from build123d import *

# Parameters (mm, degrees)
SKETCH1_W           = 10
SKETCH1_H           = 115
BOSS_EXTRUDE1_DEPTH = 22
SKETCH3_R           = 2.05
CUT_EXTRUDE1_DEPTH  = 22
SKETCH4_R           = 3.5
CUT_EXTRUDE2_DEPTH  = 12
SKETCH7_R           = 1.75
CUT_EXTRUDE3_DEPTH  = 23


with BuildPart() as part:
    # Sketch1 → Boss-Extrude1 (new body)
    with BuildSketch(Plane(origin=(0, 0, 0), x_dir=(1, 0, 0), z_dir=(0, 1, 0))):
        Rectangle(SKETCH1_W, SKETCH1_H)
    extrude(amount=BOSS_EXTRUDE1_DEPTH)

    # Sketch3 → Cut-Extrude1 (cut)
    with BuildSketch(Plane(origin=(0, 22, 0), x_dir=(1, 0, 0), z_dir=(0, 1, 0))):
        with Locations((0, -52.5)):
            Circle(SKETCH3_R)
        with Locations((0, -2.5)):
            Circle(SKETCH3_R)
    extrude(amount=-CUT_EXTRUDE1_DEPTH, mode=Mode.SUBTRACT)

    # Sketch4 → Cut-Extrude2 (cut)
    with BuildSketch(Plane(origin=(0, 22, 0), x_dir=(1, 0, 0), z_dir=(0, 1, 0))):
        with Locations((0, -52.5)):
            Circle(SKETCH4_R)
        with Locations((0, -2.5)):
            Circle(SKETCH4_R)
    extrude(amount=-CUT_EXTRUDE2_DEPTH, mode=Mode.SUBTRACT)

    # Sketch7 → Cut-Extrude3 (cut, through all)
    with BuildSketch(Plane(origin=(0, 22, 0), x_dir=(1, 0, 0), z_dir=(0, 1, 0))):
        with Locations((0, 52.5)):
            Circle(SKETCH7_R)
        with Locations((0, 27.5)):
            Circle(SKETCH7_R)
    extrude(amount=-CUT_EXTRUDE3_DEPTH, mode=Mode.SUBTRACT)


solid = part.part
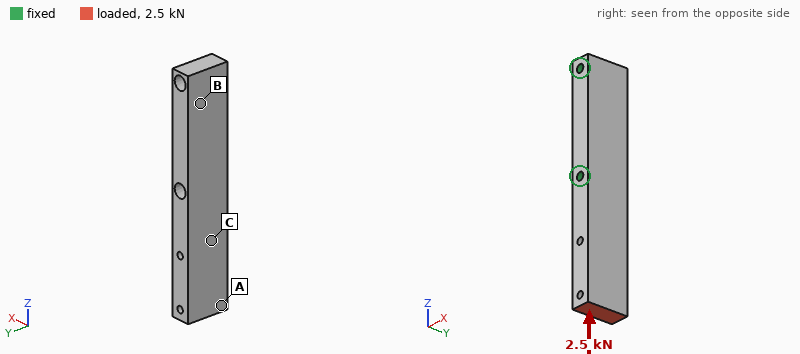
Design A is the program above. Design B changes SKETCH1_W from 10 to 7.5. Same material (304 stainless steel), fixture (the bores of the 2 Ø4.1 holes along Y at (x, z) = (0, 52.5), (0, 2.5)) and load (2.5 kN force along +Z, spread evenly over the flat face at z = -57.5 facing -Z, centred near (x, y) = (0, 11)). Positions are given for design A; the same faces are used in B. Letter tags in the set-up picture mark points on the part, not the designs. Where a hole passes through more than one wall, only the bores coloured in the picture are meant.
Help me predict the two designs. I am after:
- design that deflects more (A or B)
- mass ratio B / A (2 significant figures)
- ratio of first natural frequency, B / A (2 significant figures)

B
0.73
0.78
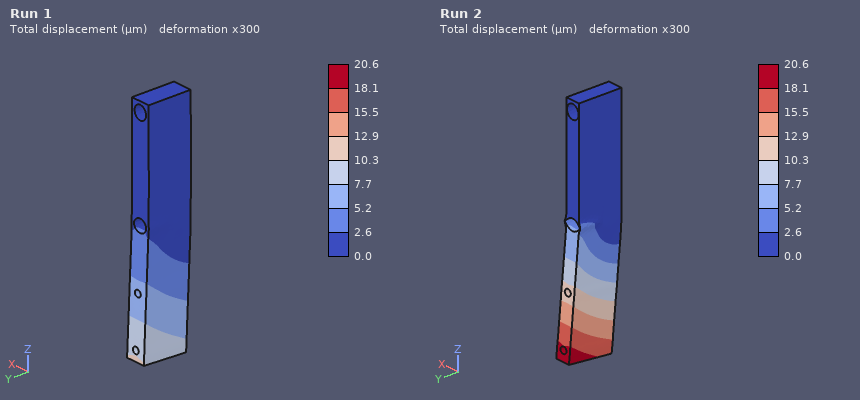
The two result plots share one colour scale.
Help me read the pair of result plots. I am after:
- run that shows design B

Run 2
